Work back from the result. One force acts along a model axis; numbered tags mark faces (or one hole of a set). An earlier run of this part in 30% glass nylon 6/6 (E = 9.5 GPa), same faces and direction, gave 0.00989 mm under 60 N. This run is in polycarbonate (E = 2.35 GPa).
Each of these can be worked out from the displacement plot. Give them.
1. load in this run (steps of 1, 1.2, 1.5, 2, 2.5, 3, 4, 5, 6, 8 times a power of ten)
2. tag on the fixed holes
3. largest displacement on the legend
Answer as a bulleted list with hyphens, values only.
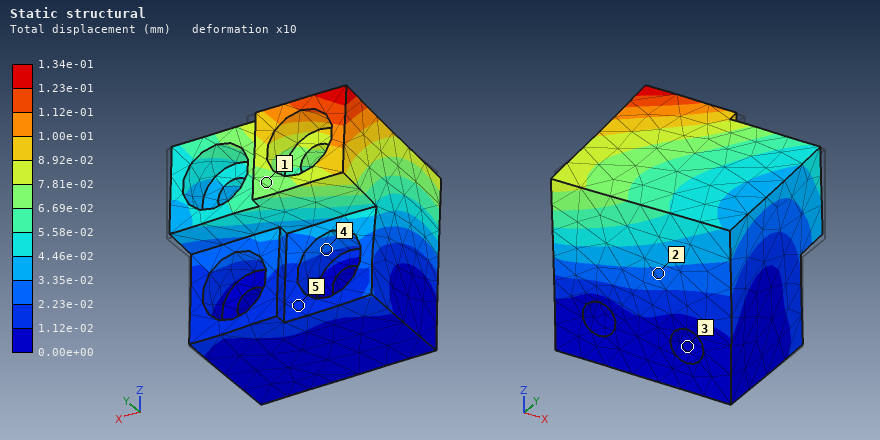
- 200 N
- 3
- 1.34e-01 mm
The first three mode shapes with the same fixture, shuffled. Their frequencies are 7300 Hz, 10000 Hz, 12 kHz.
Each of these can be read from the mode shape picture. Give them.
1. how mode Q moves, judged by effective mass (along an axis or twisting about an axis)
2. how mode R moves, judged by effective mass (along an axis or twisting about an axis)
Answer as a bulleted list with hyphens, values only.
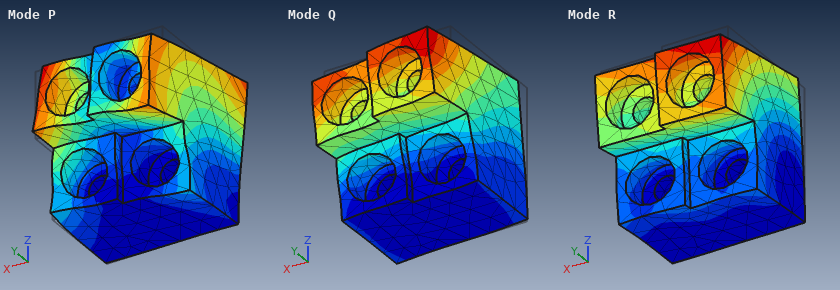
- along X
- along Y
